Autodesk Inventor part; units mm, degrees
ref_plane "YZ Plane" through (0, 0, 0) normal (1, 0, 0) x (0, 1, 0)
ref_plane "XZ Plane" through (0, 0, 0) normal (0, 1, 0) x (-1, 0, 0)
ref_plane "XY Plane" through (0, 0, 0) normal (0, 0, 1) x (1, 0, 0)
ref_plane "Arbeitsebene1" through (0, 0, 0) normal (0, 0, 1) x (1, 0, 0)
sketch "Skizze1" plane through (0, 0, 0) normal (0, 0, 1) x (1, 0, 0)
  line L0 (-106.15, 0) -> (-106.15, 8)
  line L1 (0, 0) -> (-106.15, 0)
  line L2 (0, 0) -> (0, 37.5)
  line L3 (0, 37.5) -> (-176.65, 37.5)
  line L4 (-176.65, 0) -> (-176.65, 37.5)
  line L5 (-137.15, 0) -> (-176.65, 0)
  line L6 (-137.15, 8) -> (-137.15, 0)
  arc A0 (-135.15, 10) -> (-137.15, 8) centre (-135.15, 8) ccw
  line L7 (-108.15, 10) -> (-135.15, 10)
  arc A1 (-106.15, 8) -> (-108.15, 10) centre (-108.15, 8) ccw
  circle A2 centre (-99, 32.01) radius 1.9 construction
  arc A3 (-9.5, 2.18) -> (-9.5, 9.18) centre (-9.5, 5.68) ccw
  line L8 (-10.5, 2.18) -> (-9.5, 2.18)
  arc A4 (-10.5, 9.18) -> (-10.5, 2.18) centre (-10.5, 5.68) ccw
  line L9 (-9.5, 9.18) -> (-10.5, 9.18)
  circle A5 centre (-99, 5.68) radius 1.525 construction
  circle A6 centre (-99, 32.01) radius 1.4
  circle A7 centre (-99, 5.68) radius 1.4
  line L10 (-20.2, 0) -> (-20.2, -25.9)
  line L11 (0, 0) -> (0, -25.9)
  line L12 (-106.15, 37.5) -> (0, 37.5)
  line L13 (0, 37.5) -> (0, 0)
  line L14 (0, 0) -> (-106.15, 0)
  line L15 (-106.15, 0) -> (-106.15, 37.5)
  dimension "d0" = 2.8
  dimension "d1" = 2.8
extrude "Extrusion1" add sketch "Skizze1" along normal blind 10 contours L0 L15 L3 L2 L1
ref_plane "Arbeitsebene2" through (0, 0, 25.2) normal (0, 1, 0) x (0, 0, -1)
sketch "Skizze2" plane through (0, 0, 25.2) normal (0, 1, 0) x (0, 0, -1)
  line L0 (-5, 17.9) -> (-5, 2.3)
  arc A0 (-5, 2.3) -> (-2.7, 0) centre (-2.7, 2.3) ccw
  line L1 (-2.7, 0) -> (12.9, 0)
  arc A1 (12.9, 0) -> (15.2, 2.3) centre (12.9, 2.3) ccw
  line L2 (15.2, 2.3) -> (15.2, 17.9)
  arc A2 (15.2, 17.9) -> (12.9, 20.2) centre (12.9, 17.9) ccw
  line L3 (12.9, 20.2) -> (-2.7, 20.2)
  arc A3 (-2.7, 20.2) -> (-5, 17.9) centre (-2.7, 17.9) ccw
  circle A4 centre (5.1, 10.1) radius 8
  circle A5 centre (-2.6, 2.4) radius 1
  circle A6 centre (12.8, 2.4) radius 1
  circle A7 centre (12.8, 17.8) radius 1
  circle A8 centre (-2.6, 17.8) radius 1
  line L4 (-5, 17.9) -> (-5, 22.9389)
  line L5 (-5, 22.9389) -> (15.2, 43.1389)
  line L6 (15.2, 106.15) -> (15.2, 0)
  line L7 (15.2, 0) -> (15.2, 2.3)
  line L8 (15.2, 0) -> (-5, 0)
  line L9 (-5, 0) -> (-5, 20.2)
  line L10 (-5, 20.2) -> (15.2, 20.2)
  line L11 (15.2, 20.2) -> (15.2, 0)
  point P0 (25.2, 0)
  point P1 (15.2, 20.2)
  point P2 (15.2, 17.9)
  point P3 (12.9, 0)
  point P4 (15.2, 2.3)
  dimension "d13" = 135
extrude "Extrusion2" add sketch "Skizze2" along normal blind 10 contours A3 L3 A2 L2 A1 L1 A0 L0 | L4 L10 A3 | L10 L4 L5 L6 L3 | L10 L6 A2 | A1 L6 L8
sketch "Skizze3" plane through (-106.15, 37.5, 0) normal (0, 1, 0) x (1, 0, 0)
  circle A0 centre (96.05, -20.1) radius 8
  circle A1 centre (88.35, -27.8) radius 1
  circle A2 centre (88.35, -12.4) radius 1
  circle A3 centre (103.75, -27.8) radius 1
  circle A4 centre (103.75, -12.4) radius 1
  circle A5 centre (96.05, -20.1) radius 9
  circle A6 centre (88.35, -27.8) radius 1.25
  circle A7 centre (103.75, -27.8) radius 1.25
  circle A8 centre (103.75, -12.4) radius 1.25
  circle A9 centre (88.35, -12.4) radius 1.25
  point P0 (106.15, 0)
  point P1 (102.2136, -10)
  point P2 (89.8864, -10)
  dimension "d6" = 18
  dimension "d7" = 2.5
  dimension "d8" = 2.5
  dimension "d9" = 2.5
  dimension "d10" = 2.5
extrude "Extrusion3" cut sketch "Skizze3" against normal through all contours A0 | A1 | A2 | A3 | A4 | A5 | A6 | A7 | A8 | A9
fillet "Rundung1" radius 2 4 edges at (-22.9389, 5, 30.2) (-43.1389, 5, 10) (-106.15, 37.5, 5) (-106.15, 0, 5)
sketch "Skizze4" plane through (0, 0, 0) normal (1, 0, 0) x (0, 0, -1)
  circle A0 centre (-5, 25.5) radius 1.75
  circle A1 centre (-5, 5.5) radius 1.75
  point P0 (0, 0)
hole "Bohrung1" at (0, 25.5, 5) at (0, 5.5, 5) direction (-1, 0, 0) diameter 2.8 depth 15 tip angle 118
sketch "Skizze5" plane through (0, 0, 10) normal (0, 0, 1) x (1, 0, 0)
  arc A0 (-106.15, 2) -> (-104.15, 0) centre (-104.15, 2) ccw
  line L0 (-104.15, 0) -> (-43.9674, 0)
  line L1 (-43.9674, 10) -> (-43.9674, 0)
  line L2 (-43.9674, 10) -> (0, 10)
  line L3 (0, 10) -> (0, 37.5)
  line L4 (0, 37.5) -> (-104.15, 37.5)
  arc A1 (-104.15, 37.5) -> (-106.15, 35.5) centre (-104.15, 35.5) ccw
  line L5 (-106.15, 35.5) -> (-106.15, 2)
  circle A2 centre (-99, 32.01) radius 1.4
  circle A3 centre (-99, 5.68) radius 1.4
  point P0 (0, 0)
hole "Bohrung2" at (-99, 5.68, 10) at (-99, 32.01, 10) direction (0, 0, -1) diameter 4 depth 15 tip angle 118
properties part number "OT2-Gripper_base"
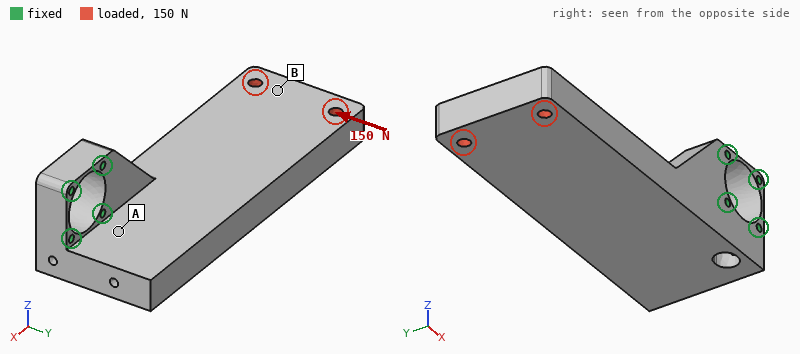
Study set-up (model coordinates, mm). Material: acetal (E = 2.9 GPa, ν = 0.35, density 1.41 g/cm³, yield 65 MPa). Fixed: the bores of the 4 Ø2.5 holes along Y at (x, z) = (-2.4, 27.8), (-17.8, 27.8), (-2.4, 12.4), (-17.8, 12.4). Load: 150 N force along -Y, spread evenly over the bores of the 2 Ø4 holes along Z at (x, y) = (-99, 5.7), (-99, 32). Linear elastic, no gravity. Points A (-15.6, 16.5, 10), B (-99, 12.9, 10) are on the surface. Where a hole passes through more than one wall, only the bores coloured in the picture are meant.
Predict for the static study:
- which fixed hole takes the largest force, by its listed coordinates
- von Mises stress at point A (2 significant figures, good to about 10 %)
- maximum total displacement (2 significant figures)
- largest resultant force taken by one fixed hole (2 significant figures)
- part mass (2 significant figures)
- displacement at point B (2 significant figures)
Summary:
(-17.8, 12.4)
5.8 MPa
1.1 mm
620 N
60 g
0.92 mm
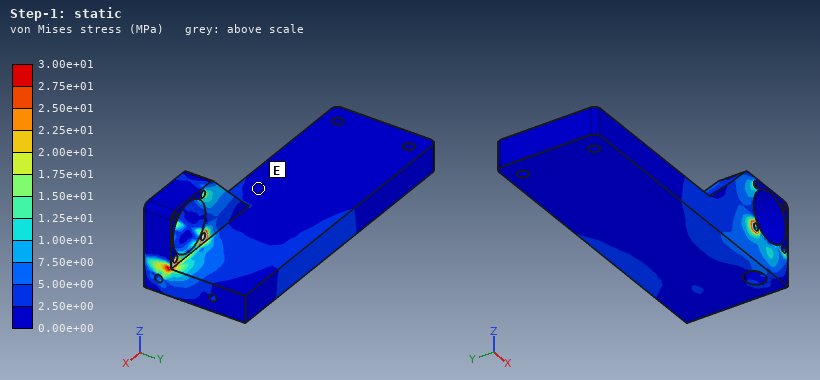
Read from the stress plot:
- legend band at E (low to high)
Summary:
0.00e+00 to 2.50e+00 MPa
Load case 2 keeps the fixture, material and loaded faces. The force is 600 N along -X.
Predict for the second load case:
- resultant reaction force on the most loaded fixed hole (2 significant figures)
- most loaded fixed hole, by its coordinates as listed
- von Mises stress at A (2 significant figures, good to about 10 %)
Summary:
570 N
(-17.8, 12.4)
3.8 MPa
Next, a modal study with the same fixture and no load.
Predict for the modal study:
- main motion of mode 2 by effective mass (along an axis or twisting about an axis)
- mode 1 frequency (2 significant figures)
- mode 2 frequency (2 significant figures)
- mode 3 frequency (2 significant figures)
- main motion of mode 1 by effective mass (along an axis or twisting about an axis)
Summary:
along Y
330 Hz
480 Hz
940 Hz
along Z
